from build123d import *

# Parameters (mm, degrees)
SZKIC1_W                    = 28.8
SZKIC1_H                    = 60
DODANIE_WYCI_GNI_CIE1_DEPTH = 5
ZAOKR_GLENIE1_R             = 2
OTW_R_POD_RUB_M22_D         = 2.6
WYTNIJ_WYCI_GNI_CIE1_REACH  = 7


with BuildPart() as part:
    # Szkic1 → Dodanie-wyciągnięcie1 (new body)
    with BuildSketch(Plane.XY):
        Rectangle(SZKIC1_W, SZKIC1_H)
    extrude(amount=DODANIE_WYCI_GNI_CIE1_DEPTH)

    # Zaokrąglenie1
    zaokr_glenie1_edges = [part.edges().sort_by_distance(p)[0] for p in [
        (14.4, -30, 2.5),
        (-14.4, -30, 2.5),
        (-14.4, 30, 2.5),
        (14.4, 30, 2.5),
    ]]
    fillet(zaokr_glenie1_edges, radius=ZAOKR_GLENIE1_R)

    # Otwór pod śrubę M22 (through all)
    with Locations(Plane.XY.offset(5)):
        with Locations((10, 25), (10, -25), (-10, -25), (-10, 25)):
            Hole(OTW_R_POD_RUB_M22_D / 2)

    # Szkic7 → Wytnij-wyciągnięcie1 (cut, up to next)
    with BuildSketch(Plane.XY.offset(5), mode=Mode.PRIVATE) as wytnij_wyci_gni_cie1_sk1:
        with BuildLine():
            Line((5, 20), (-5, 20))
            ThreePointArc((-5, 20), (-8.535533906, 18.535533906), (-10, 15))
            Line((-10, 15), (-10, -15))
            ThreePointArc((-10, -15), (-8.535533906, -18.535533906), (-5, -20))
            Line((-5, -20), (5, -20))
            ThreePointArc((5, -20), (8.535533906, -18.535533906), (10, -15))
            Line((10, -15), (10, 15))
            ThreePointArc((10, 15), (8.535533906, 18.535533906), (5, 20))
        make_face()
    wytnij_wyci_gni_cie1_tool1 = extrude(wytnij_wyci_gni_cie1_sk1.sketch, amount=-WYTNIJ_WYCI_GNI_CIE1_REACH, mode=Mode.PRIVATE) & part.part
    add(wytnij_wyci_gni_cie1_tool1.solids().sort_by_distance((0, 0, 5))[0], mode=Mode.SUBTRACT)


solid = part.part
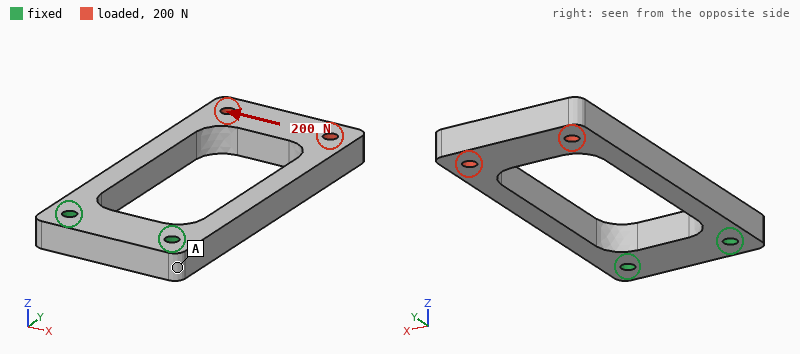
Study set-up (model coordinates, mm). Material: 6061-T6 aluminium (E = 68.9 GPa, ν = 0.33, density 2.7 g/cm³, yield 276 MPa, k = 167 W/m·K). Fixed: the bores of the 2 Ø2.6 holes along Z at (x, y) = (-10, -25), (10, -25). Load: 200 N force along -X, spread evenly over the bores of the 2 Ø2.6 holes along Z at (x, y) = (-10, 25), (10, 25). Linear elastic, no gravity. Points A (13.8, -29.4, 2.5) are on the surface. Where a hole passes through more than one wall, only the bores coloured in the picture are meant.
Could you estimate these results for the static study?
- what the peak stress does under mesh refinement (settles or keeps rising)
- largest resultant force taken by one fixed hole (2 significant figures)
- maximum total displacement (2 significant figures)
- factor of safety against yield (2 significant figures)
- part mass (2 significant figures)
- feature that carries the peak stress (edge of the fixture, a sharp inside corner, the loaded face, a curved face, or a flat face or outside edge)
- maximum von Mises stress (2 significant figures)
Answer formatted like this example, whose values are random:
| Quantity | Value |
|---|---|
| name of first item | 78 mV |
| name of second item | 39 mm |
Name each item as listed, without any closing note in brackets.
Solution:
| Quantity | Value |
|---|---|
| what the peak stress does under mesh refinement | settles |
| largest resultant force taken by one fixed hole | 420 N |
| maximum total displacement | 0.25 mm |
| factor of safety against yield | 2.4 |
| part mass | 12 g |
| feature that carries the peak stress | a curved face |
| maximum von Mises stress | 120 MPa |
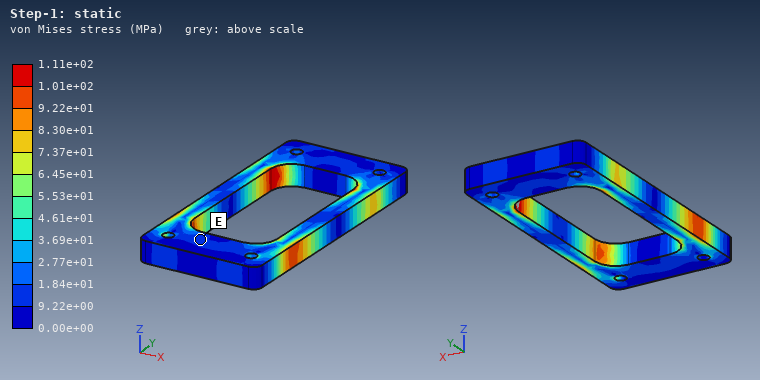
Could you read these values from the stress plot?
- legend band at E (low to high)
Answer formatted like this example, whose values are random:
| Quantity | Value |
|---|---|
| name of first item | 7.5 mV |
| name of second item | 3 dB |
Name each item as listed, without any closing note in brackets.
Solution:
| Quantity | Value |
|---|---|
| legend band at E | 9.22e+00 to 1.84e+01 MPa |
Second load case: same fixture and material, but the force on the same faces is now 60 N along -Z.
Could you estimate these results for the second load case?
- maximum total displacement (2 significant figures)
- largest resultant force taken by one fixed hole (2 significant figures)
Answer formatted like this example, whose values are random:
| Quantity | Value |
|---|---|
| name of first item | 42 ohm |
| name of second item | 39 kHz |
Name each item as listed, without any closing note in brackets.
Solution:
| Quantity | Value |
|---|---|
| maximum total displacement | 0.40 mm |
| largest resultant force taken by one fixed hole | 30 N |
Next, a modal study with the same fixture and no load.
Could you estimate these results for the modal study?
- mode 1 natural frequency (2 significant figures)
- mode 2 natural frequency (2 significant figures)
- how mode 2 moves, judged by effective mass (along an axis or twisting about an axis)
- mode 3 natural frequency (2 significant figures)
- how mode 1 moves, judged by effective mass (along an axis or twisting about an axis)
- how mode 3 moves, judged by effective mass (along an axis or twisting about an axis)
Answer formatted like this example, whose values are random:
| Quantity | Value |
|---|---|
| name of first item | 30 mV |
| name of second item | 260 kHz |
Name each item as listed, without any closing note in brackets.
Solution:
| Quantity | Value |
|---|---|
| mode 1 natural frequency | 970 Hz |
| mode 2 natural frequency | 1900 Hz |
| how mode 2 moves, judged by effective mass | along X |
| mode 3 natural frequency | 3000 Hz |
| how mode 1 moves, judged by effective mass | along Z |
| how mode 3 moves, judged by effective mass | twisting about Y |
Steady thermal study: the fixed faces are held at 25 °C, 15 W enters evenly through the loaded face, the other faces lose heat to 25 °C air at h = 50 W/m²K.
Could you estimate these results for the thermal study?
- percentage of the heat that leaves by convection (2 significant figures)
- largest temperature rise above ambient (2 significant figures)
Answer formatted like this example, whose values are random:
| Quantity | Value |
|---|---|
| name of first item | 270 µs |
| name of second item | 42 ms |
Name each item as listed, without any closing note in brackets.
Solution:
| Quantity | Value |
|---|---|
| percentage of the heat that leaves by convection | 34 % |
| largest temperature rise above ambient | 66 K |
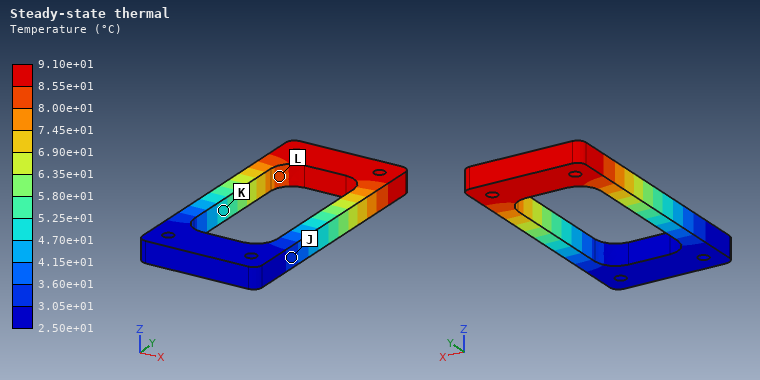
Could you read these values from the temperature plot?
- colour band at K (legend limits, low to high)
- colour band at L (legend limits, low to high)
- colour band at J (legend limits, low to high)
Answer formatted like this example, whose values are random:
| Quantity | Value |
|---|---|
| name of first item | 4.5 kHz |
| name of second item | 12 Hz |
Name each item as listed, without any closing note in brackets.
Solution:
| Quantity | Value |
|---|---|
| colour band at K | 4.70e+01 to 5.25e+01 °C |
| colour band at L | 8.00e+01 to 8.55e+01 °C |
| colour band at J | 3.05e+01 to 3.60e+01 °C |
